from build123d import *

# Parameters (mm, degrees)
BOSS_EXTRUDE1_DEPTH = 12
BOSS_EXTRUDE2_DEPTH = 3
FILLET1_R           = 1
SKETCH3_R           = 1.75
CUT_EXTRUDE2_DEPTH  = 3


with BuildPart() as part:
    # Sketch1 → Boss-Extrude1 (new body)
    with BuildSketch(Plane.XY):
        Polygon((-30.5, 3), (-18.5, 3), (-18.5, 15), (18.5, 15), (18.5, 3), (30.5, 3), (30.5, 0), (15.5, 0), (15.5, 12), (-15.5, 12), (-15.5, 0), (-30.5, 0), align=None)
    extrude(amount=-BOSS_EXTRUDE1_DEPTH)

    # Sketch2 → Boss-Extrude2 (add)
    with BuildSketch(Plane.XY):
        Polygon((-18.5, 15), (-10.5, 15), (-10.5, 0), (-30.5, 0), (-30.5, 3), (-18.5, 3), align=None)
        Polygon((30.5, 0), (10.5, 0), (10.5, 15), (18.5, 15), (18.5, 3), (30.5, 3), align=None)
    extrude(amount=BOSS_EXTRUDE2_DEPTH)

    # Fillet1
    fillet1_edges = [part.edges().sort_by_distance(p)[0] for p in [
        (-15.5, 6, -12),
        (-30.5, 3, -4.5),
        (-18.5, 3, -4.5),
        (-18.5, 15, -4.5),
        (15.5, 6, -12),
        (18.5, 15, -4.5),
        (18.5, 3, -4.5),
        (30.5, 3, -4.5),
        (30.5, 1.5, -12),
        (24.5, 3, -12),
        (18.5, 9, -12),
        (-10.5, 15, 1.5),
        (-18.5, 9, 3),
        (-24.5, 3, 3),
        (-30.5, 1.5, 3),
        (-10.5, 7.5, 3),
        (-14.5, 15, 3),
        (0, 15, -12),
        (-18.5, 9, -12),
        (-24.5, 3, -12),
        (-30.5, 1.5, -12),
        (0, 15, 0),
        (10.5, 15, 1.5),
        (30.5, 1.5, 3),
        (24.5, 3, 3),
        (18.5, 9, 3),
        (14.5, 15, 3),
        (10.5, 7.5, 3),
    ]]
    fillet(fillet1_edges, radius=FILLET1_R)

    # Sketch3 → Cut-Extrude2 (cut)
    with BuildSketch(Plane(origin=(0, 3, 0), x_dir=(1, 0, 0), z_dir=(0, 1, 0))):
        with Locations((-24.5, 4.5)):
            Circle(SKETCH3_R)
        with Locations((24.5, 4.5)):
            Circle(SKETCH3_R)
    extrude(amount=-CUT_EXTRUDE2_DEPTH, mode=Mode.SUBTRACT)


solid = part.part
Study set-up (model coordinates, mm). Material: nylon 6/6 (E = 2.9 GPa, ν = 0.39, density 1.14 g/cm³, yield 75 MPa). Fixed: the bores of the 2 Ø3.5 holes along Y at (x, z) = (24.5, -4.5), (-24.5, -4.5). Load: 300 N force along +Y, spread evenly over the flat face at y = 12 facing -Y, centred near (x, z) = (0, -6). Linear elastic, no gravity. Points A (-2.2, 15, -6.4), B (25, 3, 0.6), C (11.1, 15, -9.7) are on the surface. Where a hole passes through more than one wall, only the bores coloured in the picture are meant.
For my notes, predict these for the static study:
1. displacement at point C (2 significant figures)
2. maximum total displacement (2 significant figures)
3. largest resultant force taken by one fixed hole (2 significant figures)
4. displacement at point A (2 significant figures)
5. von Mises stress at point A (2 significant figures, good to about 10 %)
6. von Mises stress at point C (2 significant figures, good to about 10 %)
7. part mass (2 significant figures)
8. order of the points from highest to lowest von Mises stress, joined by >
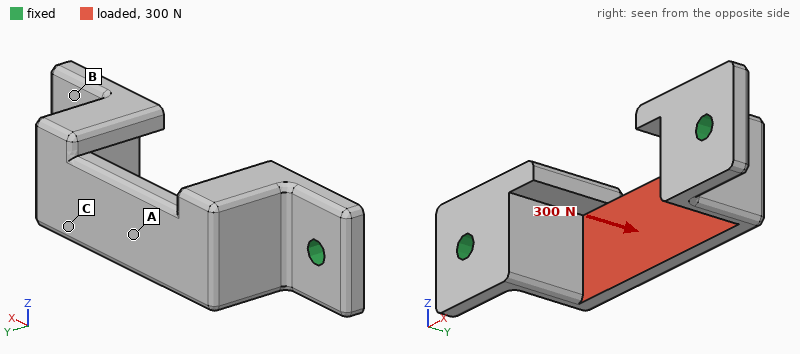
0.34 mm
0.68 mm
190 N
0.52 mm
24 MPa
11 MPa
4.4 g
A > C > B
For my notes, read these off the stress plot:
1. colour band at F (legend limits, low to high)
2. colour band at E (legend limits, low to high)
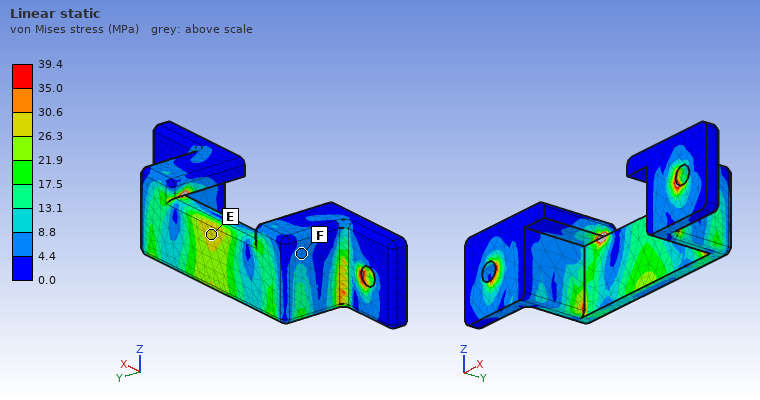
4.4 to 8.8 MPa
26.3 to 30.6 MPa
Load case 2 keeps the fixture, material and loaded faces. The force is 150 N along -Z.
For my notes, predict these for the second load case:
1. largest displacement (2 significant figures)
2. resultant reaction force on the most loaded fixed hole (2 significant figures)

0.51 mm
75 N
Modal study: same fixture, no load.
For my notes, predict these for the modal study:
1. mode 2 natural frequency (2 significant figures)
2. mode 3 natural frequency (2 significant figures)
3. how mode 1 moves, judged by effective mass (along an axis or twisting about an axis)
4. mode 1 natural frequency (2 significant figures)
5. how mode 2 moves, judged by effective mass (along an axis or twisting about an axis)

2300 Hz
3000 Hz
along Z
1800 Hz
along X
